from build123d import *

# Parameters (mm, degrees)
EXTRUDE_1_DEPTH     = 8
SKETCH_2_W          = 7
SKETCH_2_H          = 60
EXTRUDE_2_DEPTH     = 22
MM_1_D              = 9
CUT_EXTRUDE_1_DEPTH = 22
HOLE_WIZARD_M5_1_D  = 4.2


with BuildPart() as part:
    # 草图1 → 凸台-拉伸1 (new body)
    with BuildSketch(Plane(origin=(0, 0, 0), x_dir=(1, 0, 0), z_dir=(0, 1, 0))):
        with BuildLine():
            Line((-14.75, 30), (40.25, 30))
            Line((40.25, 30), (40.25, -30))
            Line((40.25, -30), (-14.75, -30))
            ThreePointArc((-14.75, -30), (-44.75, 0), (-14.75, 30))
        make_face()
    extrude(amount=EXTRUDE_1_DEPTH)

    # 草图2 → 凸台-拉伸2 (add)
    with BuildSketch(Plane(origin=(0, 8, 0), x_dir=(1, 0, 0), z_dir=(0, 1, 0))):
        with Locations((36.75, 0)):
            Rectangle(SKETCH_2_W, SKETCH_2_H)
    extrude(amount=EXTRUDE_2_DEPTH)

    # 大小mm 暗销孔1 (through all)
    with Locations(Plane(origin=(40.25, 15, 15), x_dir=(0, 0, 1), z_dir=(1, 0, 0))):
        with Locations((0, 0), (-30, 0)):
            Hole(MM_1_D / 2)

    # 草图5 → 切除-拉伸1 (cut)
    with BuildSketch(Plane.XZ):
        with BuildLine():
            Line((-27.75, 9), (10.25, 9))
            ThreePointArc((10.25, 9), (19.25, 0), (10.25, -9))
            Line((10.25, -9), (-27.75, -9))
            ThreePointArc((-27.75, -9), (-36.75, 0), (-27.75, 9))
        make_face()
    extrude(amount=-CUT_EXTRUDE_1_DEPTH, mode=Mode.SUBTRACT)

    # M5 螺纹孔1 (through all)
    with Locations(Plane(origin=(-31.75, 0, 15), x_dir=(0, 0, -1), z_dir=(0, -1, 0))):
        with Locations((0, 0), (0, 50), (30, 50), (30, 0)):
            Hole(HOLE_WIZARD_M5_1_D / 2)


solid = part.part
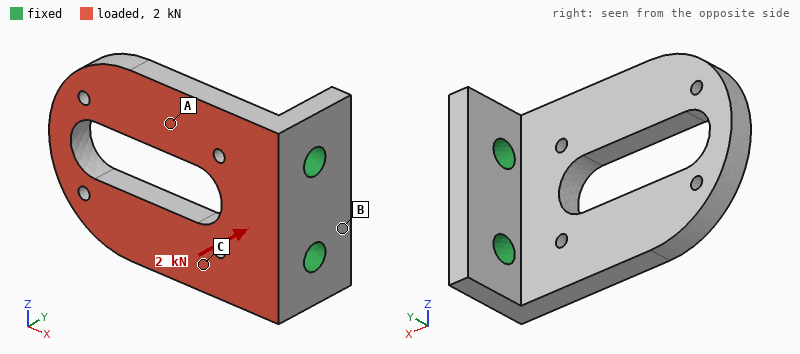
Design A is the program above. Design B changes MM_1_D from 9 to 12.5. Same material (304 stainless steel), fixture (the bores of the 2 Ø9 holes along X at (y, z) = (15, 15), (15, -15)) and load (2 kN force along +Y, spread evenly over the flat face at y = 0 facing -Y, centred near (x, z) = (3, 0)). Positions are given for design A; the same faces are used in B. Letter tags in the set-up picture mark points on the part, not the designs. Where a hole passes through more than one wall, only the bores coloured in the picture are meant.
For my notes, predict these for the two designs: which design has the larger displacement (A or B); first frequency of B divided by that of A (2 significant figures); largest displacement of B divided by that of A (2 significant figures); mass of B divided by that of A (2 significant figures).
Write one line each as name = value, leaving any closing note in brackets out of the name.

which design has the larger displacement = A
first frequency of B divided by that of A = 1.1
largest displacement of B divided by that of A = 0.90
mass of B divided by that of A = 0.98
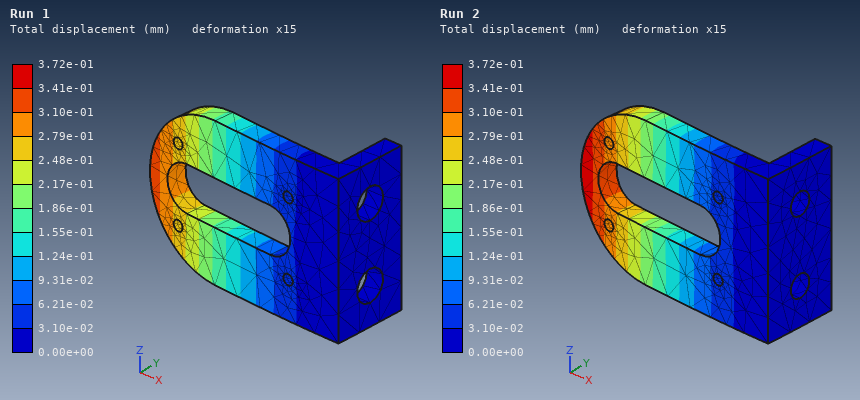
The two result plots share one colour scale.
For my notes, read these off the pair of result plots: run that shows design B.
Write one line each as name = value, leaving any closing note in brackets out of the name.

run that shows design B = Run 1
